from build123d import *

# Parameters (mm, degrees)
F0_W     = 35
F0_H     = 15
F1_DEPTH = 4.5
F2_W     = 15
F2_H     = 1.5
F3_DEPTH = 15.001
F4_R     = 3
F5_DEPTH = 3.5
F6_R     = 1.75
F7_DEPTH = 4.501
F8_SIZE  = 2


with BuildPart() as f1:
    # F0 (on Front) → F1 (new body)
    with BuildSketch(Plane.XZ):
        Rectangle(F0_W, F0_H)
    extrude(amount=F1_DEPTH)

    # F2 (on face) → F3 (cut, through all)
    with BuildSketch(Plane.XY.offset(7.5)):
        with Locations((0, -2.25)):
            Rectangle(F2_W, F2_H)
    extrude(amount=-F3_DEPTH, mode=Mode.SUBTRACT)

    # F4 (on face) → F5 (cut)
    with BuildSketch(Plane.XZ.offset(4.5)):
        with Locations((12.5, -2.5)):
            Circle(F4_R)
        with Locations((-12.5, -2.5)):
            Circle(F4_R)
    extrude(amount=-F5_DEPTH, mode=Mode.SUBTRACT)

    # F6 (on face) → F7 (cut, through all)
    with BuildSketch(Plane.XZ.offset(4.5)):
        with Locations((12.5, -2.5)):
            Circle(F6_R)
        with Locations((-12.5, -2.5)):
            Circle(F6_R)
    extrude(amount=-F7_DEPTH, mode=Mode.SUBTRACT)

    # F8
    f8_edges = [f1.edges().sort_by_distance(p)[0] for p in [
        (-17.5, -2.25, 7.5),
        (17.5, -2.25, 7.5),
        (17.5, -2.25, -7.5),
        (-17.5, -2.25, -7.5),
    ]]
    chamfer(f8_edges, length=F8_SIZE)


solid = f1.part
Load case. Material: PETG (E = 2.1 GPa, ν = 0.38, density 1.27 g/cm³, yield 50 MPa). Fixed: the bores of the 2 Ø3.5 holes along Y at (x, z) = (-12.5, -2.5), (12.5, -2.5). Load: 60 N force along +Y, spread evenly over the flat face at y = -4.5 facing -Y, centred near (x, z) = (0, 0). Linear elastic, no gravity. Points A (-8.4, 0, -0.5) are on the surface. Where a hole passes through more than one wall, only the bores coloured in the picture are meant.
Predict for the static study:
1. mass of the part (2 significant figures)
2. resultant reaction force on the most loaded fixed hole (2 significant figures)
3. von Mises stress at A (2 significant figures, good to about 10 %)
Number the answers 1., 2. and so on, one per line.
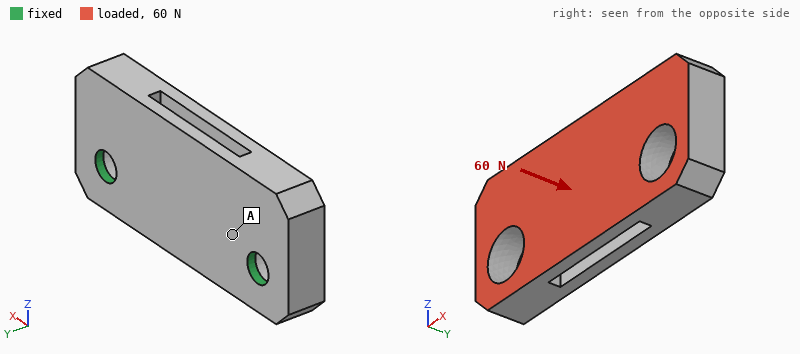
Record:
1. 2.3 g
2. 34 N
3. 2.2 MPa
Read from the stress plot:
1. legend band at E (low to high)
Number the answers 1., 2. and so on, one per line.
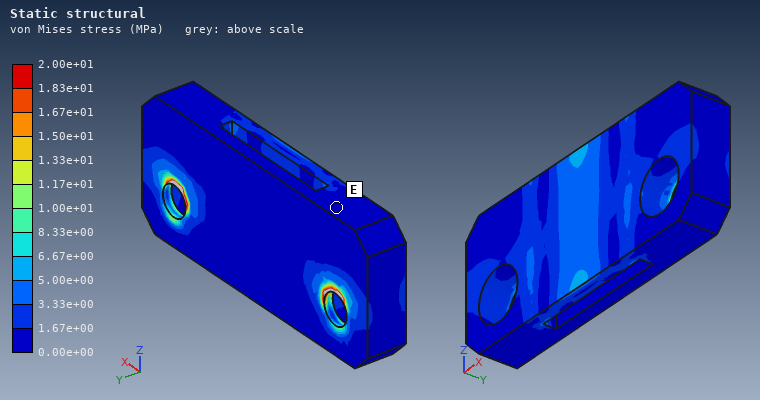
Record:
1. 0.00e+00 to 1.67e+00 MPa
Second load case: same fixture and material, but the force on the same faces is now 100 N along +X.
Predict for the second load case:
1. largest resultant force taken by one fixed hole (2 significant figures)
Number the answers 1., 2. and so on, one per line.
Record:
1. 52 N
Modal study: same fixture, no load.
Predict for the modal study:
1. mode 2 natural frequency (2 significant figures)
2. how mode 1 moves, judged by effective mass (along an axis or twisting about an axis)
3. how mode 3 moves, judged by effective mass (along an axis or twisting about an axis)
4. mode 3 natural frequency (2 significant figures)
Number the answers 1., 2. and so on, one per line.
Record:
1. 4200 Hz
2. along Y
3. along Y
4. 5200 Hz
